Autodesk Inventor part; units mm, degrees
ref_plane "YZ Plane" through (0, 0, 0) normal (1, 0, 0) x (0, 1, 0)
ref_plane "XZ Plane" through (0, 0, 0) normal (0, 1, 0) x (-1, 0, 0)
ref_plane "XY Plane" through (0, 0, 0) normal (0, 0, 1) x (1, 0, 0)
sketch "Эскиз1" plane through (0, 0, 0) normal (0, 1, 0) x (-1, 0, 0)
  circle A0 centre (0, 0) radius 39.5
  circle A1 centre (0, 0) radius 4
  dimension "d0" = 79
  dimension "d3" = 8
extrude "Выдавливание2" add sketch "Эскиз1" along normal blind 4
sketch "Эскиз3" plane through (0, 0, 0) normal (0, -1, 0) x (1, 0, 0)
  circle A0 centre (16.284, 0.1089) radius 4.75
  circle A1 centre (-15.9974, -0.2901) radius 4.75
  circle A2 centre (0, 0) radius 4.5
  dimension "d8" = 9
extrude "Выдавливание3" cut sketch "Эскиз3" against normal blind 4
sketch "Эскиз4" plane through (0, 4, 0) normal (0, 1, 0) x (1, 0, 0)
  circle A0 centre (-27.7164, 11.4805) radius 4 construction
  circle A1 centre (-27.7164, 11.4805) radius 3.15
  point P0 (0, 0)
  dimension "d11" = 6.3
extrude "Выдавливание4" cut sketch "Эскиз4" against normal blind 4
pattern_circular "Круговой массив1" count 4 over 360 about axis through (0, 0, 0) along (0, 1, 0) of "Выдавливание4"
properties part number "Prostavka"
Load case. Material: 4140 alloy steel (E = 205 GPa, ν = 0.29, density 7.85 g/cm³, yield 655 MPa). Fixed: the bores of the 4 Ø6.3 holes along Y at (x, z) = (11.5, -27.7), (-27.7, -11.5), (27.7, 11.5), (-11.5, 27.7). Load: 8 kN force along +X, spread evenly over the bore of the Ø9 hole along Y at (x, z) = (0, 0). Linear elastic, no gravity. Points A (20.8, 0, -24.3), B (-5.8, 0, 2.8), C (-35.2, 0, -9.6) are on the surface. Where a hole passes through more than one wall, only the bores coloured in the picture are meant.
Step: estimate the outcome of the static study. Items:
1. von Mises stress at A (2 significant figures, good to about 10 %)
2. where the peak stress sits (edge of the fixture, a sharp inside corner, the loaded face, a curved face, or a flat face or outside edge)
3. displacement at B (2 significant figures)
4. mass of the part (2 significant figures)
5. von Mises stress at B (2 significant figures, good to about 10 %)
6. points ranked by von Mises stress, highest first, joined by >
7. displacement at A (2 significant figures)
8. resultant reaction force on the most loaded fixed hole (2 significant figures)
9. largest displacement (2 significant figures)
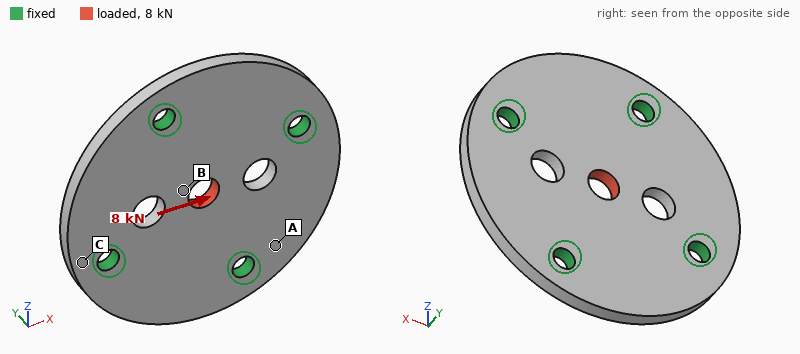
19 MPa
a curved face
6.9 µm
140 g
67 MPa
B > A > C
1.3 µm
2.4 kN
7.9 µm
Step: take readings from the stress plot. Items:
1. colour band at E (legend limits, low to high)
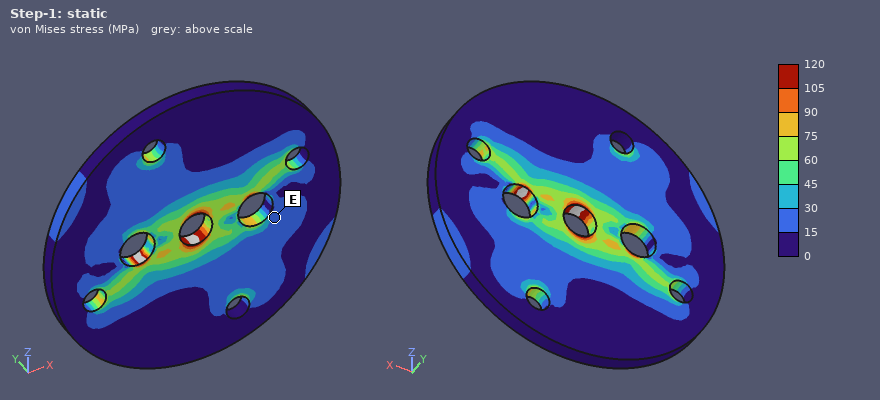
15 to 30 MPa
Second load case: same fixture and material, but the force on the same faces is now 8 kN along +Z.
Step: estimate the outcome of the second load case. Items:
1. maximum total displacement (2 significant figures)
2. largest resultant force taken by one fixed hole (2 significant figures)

6.3 µm
2.6 kN
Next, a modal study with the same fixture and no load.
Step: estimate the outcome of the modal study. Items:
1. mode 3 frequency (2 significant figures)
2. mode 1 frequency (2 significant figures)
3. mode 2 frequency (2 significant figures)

8900 Hz
8600 Hz
8800 Hz
